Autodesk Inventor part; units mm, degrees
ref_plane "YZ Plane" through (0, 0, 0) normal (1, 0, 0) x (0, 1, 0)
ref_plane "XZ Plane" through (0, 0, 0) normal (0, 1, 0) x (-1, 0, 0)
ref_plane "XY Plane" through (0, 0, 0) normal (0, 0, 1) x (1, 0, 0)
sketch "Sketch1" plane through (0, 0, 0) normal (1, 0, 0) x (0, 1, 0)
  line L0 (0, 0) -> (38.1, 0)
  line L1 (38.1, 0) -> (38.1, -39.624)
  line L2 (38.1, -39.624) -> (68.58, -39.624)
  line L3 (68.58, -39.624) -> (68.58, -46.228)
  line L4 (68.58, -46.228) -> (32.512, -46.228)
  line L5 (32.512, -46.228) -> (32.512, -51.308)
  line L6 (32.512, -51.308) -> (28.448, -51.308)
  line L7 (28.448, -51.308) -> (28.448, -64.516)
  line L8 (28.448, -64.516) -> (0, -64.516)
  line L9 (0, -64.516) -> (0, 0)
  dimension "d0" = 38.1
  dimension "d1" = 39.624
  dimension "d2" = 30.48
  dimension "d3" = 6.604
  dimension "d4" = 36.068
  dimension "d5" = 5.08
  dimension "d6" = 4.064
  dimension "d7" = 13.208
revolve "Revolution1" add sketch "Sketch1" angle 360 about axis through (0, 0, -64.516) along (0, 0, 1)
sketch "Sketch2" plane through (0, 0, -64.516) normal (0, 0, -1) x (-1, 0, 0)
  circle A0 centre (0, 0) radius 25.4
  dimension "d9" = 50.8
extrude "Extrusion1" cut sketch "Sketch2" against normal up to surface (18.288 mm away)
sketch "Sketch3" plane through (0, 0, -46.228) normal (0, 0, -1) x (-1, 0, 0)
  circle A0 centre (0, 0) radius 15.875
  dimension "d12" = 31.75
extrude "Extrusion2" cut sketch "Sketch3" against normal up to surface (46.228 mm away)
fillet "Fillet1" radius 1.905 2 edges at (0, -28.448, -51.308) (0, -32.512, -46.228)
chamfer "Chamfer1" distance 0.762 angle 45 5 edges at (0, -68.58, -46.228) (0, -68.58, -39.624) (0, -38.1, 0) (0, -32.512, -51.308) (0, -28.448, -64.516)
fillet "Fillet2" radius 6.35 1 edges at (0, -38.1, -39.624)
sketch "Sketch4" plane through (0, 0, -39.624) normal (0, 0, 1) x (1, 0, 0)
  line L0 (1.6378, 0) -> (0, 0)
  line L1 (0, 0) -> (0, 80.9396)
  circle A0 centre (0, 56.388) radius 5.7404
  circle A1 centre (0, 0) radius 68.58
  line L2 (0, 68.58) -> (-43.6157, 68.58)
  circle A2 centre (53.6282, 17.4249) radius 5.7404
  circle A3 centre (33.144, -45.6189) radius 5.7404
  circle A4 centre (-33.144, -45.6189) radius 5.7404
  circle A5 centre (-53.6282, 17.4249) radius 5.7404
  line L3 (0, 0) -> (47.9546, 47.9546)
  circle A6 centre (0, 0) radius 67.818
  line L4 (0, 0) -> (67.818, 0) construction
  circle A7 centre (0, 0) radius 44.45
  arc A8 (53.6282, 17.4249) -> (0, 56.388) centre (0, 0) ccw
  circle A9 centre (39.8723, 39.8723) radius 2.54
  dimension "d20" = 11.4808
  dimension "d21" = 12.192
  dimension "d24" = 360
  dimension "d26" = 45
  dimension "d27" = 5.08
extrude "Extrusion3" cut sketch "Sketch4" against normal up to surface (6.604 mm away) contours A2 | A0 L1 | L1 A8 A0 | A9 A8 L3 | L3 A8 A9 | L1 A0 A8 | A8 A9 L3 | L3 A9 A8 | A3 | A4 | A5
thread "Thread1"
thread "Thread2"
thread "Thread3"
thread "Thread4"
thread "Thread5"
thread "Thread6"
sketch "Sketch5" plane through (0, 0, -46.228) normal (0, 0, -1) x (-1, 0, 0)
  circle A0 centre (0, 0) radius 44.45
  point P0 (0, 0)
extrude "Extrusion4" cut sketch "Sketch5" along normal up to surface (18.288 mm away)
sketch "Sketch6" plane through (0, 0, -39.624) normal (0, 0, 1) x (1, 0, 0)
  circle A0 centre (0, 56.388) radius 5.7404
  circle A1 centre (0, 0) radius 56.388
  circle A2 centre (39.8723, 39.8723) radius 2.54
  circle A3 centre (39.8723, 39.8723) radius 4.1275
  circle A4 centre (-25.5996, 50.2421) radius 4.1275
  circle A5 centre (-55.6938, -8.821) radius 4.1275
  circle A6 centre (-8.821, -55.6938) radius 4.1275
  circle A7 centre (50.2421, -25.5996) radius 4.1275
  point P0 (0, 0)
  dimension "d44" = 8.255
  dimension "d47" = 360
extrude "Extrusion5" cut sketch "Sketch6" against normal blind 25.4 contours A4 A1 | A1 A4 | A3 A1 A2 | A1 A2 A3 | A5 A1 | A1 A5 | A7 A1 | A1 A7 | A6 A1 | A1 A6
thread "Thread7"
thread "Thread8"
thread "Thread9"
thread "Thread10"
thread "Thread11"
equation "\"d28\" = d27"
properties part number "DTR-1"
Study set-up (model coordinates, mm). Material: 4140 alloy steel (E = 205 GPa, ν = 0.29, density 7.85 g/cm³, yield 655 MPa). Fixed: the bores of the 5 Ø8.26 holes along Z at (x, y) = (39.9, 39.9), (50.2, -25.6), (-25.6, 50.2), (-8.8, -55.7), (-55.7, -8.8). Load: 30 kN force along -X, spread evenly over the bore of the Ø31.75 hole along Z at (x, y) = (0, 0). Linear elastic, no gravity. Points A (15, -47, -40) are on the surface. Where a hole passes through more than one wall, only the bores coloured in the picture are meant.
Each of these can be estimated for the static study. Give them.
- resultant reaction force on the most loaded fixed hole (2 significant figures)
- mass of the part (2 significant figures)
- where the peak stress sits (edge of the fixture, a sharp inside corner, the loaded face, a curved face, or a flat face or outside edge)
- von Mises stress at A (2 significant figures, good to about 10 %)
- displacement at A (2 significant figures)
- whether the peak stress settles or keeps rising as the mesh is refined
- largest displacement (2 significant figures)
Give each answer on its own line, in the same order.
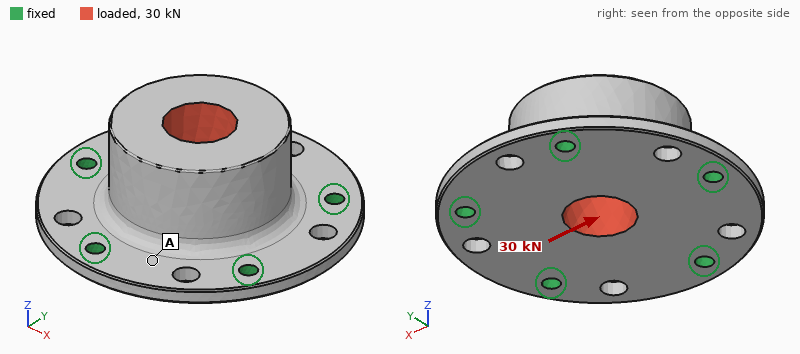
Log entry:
9.6 kN
1.9 kg
edge of the fixture
17 MPa
5.6 µm
keeps rising
28 µm
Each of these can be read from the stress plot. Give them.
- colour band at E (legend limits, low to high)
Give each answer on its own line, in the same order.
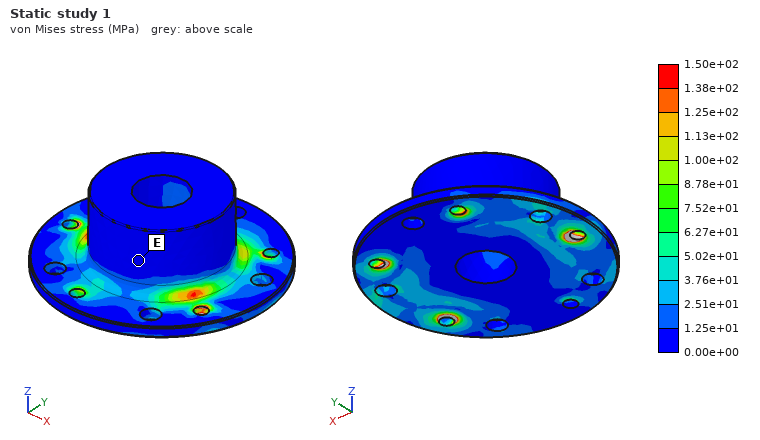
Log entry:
0.00e+00 to 1.25e+01 MPa
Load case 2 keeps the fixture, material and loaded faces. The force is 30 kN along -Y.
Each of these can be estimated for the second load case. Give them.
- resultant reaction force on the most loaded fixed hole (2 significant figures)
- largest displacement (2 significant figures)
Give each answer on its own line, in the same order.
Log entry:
9.6 kN
28 µm
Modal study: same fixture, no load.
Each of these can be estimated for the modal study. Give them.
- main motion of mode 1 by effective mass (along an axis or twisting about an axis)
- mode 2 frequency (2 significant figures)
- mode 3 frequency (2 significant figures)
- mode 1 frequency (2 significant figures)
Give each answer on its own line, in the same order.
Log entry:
along Z
4600 Hz
4600 Hz
4300 Hz
